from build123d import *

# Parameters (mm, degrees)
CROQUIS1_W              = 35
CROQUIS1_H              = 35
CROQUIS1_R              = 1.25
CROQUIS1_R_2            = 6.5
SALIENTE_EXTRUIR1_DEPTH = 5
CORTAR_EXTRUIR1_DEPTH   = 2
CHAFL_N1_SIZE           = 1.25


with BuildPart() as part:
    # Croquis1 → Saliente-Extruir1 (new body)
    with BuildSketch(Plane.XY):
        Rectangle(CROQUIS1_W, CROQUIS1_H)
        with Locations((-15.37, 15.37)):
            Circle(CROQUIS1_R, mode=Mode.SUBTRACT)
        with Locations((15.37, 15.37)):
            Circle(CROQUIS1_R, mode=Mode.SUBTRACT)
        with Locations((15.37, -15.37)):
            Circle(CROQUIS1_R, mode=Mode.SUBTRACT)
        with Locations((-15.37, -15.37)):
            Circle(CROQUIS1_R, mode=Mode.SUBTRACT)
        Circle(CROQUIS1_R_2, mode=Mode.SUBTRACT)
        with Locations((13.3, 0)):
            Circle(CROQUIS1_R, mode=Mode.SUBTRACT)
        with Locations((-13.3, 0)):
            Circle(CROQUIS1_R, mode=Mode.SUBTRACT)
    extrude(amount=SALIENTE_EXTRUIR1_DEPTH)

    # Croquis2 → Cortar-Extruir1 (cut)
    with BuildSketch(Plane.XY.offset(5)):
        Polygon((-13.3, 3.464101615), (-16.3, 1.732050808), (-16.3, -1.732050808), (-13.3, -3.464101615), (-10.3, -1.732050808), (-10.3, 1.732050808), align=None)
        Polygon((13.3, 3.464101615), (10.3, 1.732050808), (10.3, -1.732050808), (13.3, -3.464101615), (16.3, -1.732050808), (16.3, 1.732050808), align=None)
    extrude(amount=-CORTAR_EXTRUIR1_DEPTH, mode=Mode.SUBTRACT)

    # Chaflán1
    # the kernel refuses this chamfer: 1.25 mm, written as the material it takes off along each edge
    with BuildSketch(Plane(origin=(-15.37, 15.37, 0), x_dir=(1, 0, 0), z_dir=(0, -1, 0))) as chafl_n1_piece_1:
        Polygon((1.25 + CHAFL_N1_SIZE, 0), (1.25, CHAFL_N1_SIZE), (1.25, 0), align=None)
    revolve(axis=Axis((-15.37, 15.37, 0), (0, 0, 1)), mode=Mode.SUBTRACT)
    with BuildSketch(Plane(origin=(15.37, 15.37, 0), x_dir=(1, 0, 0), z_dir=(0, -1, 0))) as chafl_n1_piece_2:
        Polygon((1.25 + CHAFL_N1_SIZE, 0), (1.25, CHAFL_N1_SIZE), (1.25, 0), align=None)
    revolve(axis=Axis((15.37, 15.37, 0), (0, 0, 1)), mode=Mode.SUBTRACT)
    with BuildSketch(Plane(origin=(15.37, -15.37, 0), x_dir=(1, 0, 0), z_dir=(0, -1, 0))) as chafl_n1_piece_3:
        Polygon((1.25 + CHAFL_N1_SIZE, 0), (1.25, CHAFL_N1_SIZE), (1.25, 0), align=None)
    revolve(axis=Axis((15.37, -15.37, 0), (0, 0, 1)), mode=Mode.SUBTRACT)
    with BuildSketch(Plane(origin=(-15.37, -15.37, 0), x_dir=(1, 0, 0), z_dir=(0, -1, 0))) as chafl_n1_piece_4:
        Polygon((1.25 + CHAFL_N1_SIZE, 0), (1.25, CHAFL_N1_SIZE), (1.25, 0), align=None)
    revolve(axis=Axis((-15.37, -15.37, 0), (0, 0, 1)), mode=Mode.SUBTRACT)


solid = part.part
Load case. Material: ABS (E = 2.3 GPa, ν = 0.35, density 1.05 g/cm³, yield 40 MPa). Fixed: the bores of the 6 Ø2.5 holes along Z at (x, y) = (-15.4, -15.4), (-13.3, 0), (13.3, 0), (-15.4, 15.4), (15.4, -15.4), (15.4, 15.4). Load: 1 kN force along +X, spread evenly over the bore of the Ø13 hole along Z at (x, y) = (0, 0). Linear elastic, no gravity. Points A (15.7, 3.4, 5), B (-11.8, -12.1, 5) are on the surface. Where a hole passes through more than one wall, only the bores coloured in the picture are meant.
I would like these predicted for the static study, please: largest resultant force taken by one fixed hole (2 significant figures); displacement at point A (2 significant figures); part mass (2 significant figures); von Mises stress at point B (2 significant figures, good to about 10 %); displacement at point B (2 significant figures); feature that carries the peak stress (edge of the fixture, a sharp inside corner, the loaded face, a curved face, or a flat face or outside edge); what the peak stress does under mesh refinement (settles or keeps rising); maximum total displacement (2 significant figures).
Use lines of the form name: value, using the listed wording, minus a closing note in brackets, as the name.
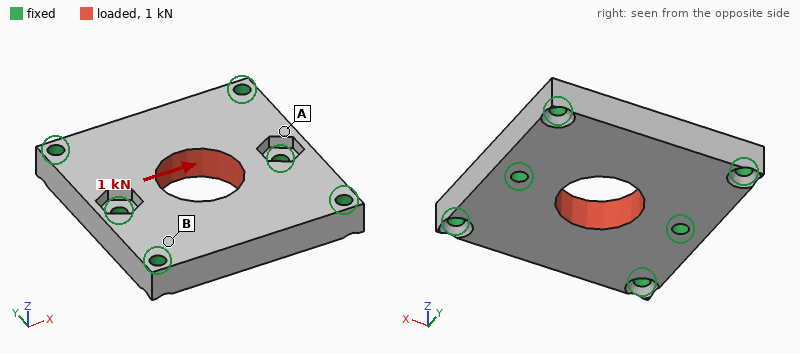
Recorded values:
largest resultant force taken by one fixed hole: 260 N
displacement at point A: 17 µm
part mass: 5.4 g
von Mises stress at point B: 5.1 MPa
displacement at point B: 10 µm
feature that carries the peak stress: edge of the fixture
what the peak stress does under mesh refinement: keeps rising
maximum total displacement: 35 µm
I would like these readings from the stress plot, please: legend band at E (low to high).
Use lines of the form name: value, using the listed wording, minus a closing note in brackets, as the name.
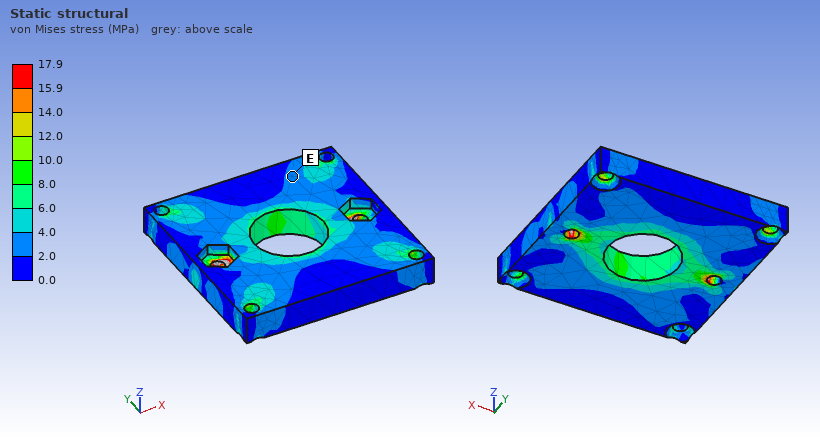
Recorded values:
legend band at E: 2.0 to 4.0 MPa
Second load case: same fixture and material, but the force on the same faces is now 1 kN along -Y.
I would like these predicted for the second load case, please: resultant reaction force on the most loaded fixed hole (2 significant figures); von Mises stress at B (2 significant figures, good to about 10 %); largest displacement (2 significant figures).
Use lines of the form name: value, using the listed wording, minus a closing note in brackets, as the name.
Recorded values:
resultant reaction force on the most loaded fixed hole: 250 N
von Mises stress at B: 6.1 MPa
largest displacement: 59 µm
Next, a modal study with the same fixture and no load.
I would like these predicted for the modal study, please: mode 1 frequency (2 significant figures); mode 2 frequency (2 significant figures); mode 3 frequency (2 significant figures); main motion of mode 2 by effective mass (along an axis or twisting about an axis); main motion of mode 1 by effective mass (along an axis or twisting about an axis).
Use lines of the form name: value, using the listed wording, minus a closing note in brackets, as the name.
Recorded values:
mode 1 frequency: 6200 Hz
mode 2 frequency: 6700 Hz
mode 3 frequency: 12 kHz
main motion of mode 2 by effective mass: twisting about X
main motion of mode 1 by effective mass: along Z
